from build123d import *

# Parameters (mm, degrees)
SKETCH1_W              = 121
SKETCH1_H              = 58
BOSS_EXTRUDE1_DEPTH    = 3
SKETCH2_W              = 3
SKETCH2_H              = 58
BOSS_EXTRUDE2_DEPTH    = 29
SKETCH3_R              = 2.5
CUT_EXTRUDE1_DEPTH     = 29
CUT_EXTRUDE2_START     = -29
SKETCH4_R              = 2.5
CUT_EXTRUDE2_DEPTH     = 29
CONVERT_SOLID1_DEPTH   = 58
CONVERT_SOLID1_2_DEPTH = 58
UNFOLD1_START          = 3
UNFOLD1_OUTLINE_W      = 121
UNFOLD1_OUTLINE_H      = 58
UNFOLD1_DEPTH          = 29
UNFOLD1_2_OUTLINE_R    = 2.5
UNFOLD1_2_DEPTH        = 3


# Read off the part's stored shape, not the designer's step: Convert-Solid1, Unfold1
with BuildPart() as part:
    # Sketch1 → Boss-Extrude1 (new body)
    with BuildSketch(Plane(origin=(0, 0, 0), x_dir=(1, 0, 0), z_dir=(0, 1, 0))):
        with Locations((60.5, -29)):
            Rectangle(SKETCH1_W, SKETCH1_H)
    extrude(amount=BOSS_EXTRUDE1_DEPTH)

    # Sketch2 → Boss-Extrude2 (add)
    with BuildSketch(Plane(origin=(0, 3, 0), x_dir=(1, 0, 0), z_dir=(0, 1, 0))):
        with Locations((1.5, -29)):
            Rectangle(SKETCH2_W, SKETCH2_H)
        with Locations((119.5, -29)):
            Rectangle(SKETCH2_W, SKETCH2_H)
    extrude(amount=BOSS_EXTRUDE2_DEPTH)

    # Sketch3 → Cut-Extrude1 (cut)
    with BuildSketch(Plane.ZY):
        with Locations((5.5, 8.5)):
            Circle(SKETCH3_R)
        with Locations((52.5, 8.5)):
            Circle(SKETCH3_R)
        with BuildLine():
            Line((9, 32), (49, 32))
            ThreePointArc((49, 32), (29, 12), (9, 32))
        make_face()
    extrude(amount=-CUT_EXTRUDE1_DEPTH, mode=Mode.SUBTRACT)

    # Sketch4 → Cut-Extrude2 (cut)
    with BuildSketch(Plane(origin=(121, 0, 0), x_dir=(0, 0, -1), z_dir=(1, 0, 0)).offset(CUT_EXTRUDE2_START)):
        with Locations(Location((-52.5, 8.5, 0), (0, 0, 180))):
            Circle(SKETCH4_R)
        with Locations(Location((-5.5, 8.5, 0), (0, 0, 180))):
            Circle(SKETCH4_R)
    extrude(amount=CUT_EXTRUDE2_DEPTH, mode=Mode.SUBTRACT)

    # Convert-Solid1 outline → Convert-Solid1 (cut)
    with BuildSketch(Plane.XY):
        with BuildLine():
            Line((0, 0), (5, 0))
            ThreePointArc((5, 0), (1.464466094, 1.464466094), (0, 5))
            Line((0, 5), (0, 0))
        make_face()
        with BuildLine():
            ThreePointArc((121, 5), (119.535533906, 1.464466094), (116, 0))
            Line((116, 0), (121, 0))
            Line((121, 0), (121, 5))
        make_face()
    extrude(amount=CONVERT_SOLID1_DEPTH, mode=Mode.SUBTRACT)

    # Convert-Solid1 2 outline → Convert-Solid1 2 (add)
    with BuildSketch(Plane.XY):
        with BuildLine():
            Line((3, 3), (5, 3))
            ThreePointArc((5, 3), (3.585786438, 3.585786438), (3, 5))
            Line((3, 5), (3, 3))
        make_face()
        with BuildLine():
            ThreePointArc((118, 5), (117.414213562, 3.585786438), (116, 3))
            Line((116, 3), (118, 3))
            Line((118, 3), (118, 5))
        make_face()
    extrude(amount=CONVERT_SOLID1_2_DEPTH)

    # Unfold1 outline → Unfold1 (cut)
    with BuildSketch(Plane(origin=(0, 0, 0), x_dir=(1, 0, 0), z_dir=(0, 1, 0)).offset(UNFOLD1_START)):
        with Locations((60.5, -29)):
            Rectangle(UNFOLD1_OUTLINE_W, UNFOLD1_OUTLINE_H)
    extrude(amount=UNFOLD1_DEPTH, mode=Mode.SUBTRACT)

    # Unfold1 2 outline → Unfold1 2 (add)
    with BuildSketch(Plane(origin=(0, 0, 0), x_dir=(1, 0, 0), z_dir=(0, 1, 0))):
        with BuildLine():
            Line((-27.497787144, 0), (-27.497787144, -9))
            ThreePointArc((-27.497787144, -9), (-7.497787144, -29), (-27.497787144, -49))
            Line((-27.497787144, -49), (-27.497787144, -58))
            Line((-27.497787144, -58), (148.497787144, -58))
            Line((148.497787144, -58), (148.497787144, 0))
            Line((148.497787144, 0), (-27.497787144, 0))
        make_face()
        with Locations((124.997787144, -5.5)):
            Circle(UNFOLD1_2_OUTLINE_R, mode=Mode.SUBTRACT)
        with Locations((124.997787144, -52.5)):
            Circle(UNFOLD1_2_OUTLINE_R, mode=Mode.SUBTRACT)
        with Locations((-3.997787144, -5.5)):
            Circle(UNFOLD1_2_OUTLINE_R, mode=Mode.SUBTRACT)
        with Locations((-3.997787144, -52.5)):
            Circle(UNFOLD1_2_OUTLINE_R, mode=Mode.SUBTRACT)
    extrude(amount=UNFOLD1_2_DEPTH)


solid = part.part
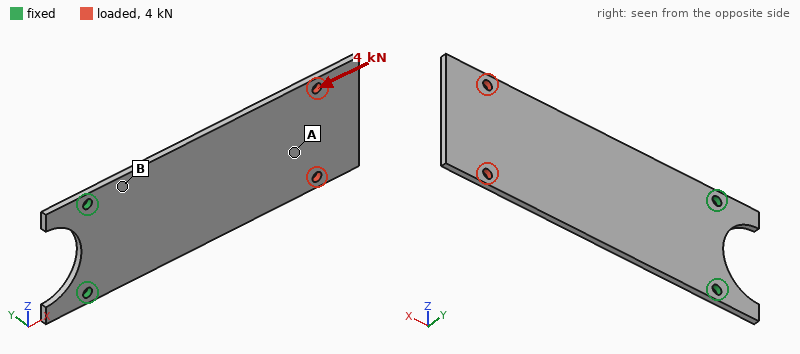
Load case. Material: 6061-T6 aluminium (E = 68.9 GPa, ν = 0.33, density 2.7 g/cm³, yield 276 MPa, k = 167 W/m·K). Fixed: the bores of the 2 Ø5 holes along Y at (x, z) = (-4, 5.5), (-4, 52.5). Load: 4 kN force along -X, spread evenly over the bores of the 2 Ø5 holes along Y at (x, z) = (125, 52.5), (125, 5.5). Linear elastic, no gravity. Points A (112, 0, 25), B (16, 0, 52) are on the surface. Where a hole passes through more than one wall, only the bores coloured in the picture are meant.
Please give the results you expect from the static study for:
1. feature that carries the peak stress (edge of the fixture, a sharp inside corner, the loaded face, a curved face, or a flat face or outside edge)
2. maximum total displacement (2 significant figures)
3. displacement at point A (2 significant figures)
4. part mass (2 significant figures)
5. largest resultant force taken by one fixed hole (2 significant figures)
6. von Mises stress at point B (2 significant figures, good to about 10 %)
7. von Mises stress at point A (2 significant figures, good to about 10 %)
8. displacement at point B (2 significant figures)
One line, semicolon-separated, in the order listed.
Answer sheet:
edge of the fixture; 55 µm; 42 µm; 77 g; 2.1 kN; 31 MPa; 14 MPa; 11 µm
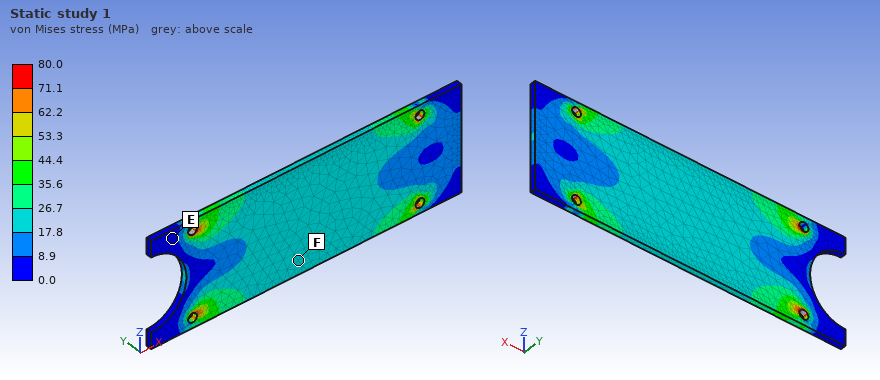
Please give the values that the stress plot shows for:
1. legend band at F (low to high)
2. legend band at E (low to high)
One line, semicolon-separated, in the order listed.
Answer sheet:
17.8 to 26.7 MPa; 0.0 to 8.9 MPa
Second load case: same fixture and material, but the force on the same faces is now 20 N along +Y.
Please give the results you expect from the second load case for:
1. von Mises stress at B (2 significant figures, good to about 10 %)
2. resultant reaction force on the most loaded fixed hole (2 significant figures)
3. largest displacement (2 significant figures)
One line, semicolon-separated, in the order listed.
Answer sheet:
26 MPa; 10 N; 2.1 mm
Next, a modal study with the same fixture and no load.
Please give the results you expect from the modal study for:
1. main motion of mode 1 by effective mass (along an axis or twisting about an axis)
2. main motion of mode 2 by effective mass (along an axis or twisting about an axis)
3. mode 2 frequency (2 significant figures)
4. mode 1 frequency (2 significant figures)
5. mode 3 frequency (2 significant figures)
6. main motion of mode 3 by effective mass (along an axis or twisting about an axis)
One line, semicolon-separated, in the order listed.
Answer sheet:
along Y; twisting about X; 580 Hz; 100 Hz; 650 Hz; along Y
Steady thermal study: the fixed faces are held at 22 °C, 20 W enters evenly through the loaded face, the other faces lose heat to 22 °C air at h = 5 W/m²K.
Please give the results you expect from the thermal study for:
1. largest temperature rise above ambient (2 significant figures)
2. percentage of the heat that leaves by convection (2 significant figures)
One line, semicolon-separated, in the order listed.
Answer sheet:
84 K; 21 %
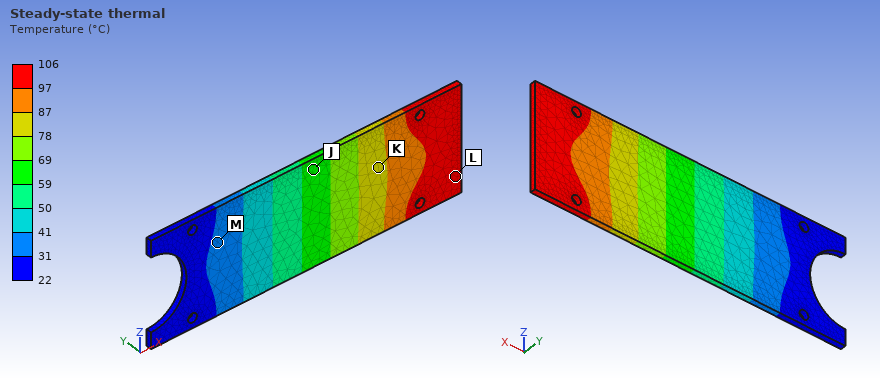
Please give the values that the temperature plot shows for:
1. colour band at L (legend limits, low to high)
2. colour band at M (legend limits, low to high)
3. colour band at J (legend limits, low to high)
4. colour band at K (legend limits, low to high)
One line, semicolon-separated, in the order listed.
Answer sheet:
97 to 106 °C; 31 to 41 °C; 59 to 69 °C; 78 to 87 °C
